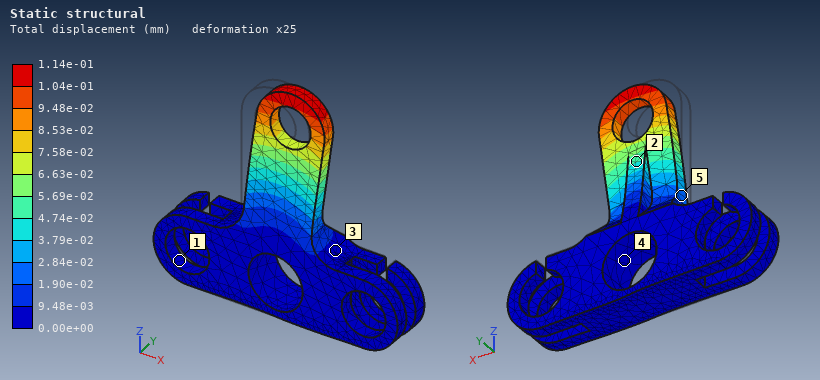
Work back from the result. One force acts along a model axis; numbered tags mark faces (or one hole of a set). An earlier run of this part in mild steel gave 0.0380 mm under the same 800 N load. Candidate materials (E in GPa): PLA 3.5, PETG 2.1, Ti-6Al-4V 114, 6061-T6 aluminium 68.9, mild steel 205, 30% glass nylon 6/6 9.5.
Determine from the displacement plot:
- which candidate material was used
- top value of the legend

6061-T6 aluminium
1.14e-01 mm
